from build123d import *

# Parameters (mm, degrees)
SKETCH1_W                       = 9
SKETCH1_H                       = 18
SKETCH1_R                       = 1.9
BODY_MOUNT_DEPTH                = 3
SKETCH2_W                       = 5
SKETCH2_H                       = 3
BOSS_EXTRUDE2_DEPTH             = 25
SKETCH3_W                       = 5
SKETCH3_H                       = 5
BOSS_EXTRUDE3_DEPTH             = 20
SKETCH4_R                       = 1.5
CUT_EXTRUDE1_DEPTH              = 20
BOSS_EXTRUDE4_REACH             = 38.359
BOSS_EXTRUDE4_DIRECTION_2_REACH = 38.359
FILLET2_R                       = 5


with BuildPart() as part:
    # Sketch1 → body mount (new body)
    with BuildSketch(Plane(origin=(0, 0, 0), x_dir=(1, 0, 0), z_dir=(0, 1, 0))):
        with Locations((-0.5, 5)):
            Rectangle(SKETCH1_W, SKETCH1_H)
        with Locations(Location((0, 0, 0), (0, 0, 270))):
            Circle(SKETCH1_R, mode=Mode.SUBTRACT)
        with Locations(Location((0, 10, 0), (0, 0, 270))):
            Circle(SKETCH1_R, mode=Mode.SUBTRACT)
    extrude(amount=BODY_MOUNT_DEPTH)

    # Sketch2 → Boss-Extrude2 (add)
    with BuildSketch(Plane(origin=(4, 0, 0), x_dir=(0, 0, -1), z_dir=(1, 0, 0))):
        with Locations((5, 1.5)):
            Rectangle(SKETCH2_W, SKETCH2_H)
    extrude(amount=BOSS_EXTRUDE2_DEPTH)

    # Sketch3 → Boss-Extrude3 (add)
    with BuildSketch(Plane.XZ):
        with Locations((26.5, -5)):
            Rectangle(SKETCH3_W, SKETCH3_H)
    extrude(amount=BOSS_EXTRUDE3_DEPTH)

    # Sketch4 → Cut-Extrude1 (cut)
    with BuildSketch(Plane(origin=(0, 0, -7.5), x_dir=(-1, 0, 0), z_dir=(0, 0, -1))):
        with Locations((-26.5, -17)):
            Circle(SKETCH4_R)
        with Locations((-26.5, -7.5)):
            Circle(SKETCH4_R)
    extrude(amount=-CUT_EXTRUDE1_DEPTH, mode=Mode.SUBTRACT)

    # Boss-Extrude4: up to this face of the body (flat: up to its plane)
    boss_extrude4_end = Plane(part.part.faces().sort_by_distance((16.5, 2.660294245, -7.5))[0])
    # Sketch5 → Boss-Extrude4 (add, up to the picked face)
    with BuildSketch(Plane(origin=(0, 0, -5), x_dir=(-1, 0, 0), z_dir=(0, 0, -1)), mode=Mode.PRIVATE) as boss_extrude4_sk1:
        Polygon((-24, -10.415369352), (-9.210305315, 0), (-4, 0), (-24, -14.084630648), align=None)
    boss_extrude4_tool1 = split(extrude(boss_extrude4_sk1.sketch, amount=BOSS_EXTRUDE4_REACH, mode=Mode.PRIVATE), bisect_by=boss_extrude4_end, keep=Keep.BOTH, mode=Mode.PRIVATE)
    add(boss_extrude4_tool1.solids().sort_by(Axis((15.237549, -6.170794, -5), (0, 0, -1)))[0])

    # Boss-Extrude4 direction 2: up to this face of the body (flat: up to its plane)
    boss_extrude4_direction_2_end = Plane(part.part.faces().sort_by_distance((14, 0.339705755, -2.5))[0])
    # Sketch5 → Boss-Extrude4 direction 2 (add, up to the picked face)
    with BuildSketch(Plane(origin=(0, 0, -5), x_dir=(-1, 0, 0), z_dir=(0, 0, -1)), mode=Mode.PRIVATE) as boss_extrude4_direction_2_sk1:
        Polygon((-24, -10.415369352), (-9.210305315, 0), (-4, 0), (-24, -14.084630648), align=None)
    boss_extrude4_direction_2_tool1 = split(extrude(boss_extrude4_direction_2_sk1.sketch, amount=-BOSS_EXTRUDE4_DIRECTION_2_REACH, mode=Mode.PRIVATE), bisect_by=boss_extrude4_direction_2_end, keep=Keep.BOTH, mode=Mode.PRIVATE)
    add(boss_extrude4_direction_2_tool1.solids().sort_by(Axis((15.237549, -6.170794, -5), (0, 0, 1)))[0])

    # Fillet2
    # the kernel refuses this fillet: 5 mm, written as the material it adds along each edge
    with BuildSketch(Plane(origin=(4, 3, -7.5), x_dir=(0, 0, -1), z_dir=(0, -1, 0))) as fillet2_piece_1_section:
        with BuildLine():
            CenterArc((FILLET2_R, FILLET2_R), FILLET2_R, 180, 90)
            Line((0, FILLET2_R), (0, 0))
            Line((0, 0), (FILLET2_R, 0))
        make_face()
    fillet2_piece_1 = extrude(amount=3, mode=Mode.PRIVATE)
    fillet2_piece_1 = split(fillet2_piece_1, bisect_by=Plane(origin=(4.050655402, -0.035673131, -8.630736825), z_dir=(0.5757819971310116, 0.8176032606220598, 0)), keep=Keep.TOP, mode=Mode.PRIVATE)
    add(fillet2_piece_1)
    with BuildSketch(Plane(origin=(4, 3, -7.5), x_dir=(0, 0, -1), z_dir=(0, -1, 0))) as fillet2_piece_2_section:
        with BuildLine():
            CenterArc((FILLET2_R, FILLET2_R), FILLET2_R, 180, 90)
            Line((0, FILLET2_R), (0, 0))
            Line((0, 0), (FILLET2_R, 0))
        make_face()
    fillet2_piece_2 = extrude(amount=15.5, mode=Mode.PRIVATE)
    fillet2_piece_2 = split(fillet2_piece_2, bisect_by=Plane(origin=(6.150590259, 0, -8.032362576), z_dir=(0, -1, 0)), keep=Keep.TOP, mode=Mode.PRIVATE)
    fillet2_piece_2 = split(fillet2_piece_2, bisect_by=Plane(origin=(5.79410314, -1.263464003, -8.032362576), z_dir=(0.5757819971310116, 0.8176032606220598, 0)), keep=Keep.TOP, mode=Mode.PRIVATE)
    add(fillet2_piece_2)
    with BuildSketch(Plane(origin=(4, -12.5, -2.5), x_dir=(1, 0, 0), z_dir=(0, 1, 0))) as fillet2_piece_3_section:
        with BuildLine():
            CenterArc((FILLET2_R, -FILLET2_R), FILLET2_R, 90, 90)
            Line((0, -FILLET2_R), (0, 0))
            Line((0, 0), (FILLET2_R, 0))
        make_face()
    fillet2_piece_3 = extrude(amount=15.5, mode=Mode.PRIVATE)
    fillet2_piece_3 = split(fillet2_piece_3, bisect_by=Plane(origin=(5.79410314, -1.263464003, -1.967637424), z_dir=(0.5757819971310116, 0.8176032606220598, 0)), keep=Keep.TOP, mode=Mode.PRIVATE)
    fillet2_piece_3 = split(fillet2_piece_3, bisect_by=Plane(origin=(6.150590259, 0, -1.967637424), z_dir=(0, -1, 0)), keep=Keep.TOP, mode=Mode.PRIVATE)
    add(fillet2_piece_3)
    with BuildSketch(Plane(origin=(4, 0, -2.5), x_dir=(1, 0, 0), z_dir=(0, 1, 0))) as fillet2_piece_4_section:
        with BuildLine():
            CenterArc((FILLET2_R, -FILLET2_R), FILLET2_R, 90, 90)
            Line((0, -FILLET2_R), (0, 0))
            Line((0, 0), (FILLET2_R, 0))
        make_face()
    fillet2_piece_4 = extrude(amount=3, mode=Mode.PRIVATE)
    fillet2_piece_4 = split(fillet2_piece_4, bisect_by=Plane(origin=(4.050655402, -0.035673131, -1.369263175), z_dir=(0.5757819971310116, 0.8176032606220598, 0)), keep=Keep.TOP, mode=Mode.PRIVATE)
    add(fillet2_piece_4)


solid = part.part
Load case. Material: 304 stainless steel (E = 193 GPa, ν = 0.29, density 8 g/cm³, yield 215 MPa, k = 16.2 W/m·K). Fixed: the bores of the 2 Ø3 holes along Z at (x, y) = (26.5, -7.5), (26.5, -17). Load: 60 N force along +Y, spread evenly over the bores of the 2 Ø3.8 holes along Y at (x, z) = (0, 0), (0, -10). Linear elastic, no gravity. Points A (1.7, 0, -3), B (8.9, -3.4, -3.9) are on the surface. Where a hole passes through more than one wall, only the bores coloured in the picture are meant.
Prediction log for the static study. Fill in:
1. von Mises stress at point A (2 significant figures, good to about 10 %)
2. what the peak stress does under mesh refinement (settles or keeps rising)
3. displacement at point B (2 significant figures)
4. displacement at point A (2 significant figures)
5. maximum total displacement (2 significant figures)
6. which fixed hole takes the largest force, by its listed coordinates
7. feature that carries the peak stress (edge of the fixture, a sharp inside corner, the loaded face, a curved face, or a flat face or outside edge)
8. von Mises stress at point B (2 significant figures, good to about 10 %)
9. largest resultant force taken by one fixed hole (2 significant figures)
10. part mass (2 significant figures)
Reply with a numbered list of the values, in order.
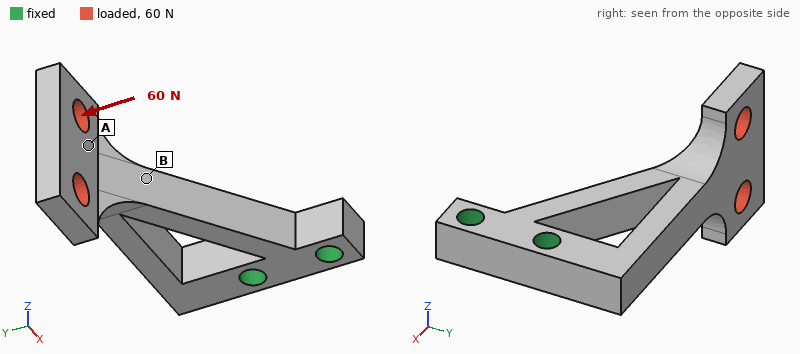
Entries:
1. 7.5 MPa
2. keeps rising
3. 4.1 µm
4. 8.8 µm
5. 15 µm
6. (26.5, -17)
7. edge of the fixture
8. 16 MPa
9. 100 N
10. 13 g
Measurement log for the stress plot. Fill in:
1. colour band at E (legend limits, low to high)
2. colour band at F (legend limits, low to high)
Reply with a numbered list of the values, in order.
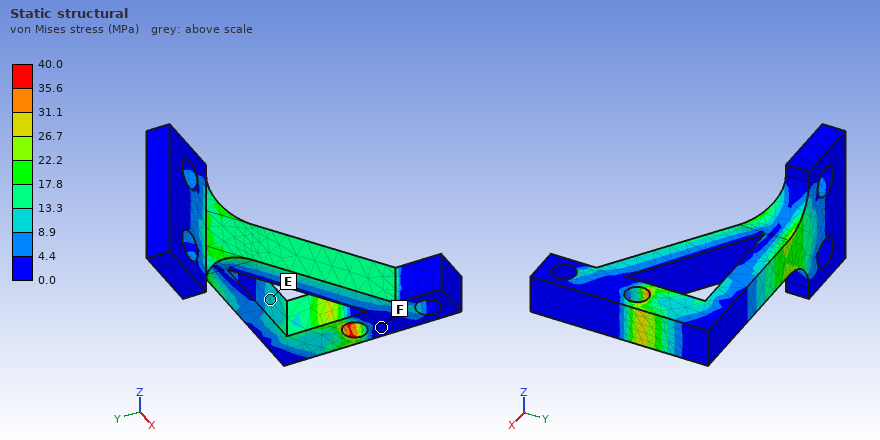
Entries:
1. 8.9 to 13.3 MPa
2. 0.0 to 4.4 MPa
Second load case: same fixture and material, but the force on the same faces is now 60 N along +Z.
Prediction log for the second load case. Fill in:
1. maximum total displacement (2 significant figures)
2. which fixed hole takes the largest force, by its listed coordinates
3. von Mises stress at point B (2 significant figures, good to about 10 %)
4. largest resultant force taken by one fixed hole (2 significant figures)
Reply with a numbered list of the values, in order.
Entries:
1. 64 µm
2. (26.5, -7.5)
3. 20 MPa
4. 87 N
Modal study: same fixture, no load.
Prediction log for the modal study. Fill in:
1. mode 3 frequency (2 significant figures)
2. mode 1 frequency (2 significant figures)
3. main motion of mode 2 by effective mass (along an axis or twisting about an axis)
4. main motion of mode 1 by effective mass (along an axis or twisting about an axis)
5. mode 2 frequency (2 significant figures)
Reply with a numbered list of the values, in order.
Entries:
1. 8700 Hz
2. 2600 Hz
3. along Y
4. along Z
5. 5400 Hz
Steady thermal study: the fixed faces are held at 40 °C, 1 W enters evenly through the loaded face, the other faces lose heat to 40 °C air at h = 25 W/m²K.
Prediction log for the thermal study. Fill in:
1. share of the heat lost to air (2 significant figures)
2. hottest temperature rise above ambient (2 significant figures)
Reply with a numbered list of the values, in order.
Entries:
1. 57 %
2. 34 K
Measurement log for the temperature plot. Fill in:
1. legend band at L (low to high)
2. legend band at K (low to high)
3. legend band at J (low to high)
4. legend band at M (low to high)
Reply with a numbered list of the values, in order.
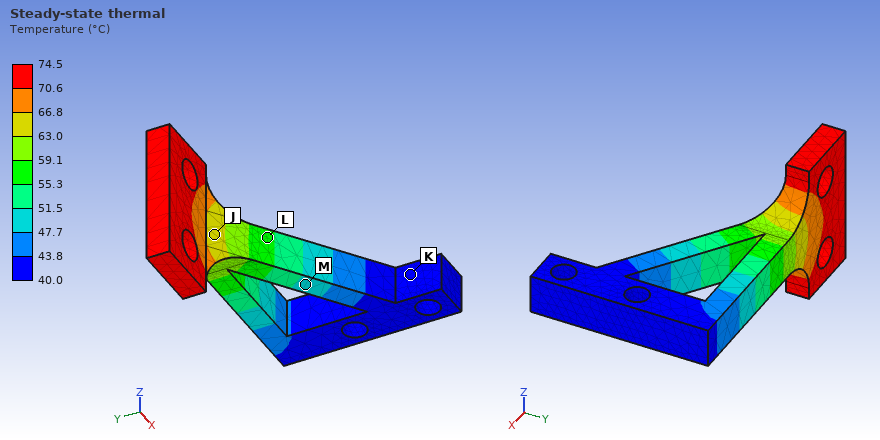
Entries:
1. 55.3 to 59.1 °C
2. 40.0 to 43.8 °C
3. 63.0 to 66.8 °C
4. 47.7 to 51.5 °C
